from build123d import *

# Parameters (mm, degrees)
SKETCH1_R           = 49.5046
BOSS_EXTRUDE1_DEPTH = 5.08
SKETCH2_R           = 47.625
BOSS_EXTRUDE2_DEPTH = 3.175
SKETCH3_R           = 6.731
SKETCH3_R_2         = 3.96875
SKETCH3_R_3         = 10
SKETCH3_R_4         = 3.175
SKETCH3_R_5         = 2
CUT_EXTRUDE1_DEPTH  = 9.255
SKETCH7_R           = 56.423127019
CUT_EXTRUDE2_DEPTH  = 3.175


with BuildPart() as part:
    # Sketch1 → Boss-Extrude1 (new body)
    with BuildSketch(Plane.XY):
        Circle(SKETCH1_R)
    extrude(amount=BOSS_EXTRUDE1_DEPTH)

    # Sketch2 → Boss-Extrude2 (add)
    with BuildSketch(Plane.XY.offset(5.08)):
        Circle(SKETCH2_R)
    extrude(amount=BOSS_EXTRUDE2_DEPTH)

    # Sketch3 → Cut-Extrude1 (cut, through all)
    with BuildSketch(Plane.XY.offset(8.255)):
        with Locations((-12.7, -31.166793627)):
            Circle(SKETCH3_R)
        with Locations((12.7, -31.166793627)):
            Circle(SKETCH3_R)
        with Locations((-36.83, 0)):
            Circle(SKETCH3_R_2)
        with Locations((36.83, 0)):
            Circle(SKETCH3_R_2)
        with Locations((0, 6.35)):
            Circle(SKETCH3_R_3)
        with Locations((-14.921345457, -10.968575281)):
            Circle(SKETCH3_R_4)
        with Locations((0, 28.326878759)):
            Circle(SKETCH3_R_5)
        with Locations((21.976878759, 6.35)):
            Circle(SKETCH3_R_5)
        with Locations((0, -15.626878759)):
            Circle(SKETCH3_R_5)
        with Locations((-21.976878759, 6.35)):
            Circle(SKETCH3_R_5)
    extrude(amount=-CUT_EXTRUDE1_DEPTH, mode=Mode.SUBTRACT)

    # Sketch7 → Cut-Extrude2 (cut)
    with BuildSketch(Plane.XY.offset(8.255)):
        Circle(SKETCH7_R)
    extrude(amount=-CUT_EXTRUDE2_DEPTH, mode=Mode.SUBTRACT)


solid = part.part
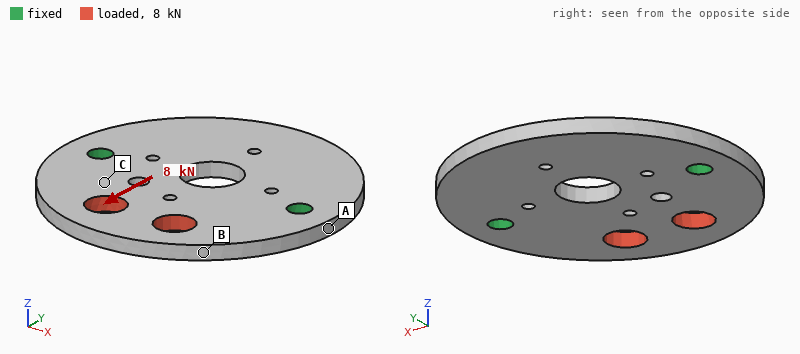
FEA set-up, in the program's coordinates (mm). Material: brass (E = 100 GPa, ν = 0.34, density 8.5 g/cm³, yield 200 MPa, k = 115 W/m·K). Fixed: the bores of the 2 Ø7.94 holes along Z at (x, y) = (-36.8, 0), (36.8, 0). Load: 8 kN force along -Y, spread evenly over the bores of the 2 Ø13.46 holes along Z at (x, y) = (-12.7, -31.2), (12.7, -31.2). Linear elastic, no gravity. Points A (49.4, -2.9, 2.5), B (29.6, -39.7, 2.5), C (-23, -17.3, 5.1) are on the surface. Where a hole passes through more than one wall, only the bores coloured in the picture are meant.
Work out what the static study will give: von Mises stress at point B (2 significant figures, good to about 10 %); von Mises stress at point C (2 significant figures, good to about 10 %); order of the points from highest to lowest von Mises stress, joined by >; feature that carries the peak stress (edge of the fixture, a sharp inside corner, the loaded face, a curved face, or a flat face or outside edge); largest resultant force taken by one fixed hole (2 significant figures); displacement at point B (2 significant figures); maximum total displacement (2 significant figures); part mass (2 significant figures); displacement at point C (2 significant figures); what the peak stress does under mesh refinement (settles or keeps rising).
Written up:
12 MPa
26 MPa
C > B > A
edge of the fixture
4.2 kN
8.8 µm
19 µm
300 g
7.8 µm
keeps rising
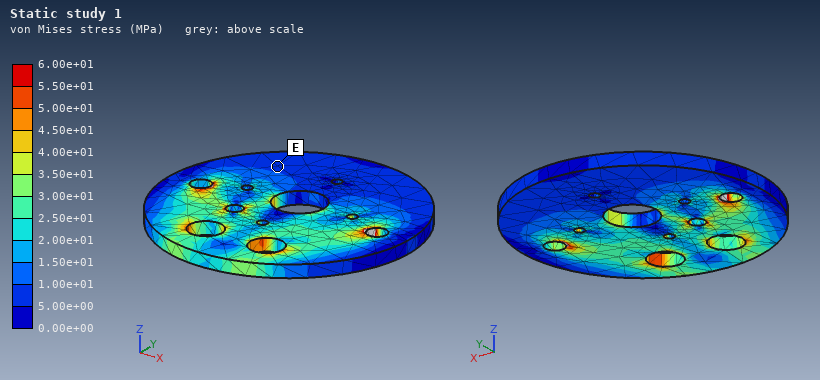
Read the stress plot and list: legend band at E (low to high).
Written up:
5.00e+00 to 1.00e+01 MPa
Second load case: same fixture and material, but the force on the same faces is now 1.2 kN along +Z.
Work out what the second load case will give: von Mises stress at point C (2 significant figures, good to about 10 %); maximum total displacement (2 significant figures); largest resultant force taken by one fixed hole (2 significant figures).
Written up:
49 MPa
0.38 mm
600 N
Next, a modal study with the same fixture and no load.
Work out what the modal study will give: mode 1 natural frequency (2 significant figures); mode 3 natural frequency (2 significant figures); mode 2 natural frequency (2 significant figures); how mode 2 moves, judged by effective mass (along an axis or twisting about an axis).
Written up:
1200 Hz
3000 Hz
1400 Hz
along Z
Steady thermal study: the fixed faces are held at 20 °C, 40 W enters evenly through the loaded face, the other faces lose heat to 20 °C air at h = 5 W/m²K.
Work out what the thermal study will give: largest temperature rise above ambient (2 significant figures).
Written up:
45 K
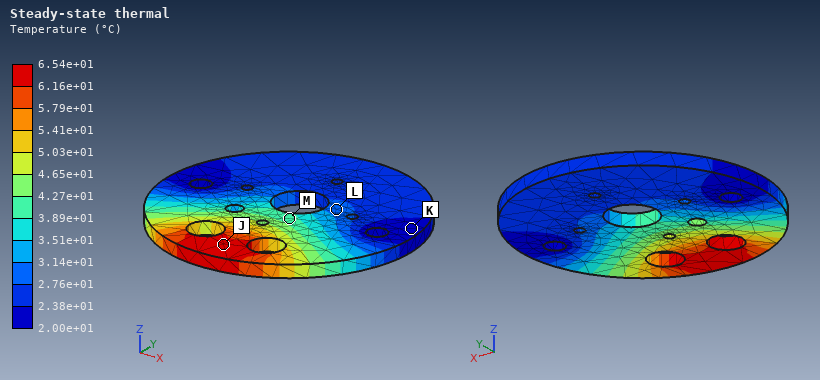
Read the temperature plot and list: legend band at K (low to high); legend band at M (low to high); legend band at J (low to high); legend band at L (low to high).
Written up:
2.00e+01 to 2.38e+01 °C
3.89e+01 to 4.27e+01 °C
6.16e+01 to 6.54e+01 °C
2.76e+01 to 3.14e+01 °C
